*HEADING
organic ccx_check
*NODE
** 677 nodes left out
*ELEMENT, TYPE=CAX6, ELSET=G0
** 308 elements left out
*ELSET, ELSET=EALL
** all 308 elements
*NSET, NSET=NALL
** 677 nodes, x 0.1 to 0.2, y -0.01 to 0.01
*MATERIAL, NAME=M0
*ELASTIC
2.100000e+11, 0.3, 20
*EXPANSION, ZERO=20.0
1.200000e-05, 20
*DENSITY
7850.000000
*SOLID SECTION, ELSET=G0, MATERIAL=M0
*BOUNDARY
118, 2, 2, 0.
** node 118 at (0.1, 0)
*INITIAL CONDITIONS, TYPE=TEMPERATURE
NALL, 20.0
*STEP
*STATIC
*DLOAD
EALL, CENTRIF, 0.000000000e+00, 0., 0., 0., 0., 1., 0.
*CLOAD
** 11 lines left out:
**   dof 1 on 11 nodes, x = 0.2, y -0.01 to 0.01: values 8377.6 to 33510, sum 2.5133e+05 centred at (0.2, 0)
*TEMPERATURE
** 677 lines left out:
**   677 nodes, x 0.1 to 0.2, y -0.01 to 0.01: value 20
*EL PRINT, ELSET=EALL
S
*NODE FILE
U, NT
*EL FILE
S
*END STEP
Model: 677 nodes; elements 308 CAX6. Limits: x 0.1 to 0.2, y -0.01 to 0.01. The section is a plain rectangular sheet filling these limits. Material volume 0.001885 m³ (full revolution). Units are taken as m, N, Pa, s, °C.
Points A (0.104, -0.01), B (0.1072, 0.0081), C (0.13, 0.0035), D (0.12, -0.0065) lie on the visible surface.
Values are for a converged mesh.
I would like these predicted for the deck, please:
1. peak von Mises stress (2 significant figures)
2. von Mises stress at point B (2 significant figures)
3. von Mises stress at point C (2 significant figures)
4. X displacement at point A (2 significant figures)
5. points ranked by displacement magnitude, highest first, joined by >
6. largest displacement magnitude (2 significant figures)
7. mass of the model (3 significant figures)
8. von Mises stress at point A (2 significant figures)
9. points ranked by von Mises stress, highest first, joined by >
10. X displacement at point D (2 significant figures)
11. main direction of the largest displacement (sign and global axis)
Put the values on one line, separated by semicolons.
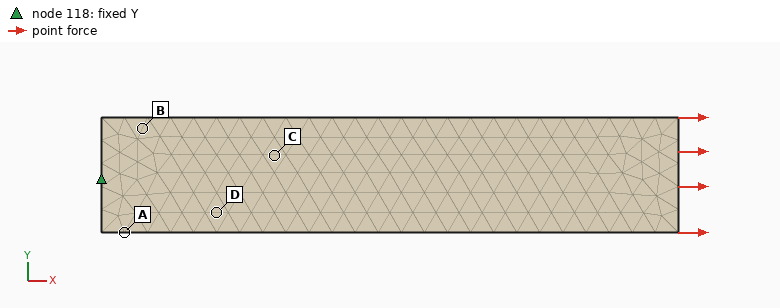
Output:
2.7e+07 Pa; 2.4e+07 Pa; 1.9e+07 Pa; 1.3e-05 m; A > B > D > C; 1.3e-05 m; 14.8 kg; 2.5e+07 Pa; A > B > D > C; 1.2e-05 m; +X
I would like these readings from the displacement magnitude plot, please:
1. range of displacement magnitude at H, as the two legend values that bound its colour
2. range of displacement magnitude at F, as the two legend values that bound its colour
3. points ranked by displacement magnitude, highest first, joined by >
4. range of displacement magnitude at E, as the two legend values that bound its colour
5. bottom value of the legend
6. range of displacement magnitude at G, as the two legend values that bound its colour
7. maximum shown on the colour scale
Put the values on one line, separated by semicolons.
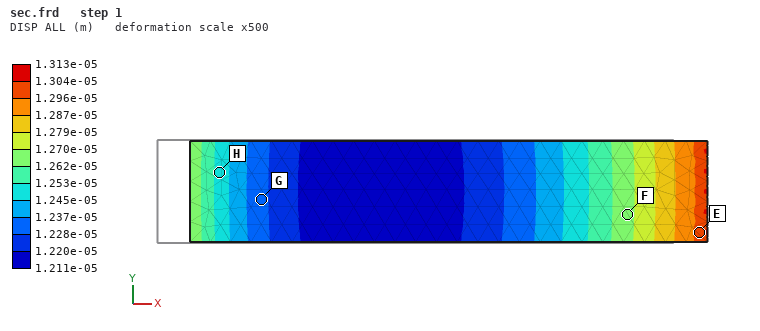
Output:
1.245e-05 to 1.253e-05 m; 1.262e-05 to 1.270e-05 m; E > F > H > G; 1.296e-05 to 1.304e-05 m; 1.211e-05 m; 1.228e-05 to 1.237e-05 m; 1.313e-05 m
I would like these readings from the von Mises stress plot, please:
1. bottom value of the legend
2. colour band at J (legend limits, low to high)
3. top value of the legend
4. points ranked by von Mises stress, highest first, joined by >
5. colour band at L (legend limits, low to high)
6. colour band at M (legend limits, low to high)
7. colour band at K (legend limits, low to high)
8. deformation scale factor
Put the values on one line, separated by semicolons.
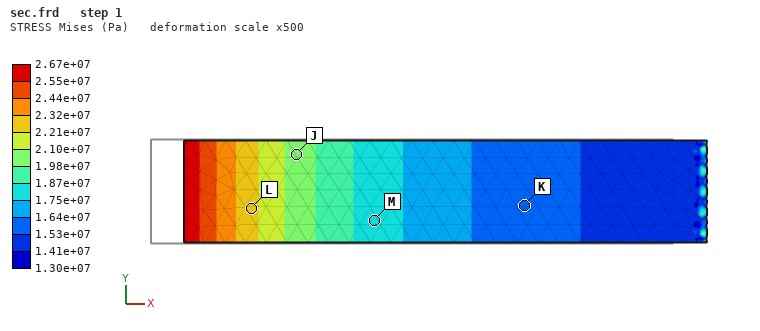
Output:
1.30e+07 Pa; 1.98e+07 to 2.10e+07 Pa; 2.67e+07 Pa; L > J > M > K; 2.21e+07 to 2.32e+07 Pa; 1.75e+07 to 1.87e+07 Pa; 1.53e+07 to 1.64e+07 Pa; 500
